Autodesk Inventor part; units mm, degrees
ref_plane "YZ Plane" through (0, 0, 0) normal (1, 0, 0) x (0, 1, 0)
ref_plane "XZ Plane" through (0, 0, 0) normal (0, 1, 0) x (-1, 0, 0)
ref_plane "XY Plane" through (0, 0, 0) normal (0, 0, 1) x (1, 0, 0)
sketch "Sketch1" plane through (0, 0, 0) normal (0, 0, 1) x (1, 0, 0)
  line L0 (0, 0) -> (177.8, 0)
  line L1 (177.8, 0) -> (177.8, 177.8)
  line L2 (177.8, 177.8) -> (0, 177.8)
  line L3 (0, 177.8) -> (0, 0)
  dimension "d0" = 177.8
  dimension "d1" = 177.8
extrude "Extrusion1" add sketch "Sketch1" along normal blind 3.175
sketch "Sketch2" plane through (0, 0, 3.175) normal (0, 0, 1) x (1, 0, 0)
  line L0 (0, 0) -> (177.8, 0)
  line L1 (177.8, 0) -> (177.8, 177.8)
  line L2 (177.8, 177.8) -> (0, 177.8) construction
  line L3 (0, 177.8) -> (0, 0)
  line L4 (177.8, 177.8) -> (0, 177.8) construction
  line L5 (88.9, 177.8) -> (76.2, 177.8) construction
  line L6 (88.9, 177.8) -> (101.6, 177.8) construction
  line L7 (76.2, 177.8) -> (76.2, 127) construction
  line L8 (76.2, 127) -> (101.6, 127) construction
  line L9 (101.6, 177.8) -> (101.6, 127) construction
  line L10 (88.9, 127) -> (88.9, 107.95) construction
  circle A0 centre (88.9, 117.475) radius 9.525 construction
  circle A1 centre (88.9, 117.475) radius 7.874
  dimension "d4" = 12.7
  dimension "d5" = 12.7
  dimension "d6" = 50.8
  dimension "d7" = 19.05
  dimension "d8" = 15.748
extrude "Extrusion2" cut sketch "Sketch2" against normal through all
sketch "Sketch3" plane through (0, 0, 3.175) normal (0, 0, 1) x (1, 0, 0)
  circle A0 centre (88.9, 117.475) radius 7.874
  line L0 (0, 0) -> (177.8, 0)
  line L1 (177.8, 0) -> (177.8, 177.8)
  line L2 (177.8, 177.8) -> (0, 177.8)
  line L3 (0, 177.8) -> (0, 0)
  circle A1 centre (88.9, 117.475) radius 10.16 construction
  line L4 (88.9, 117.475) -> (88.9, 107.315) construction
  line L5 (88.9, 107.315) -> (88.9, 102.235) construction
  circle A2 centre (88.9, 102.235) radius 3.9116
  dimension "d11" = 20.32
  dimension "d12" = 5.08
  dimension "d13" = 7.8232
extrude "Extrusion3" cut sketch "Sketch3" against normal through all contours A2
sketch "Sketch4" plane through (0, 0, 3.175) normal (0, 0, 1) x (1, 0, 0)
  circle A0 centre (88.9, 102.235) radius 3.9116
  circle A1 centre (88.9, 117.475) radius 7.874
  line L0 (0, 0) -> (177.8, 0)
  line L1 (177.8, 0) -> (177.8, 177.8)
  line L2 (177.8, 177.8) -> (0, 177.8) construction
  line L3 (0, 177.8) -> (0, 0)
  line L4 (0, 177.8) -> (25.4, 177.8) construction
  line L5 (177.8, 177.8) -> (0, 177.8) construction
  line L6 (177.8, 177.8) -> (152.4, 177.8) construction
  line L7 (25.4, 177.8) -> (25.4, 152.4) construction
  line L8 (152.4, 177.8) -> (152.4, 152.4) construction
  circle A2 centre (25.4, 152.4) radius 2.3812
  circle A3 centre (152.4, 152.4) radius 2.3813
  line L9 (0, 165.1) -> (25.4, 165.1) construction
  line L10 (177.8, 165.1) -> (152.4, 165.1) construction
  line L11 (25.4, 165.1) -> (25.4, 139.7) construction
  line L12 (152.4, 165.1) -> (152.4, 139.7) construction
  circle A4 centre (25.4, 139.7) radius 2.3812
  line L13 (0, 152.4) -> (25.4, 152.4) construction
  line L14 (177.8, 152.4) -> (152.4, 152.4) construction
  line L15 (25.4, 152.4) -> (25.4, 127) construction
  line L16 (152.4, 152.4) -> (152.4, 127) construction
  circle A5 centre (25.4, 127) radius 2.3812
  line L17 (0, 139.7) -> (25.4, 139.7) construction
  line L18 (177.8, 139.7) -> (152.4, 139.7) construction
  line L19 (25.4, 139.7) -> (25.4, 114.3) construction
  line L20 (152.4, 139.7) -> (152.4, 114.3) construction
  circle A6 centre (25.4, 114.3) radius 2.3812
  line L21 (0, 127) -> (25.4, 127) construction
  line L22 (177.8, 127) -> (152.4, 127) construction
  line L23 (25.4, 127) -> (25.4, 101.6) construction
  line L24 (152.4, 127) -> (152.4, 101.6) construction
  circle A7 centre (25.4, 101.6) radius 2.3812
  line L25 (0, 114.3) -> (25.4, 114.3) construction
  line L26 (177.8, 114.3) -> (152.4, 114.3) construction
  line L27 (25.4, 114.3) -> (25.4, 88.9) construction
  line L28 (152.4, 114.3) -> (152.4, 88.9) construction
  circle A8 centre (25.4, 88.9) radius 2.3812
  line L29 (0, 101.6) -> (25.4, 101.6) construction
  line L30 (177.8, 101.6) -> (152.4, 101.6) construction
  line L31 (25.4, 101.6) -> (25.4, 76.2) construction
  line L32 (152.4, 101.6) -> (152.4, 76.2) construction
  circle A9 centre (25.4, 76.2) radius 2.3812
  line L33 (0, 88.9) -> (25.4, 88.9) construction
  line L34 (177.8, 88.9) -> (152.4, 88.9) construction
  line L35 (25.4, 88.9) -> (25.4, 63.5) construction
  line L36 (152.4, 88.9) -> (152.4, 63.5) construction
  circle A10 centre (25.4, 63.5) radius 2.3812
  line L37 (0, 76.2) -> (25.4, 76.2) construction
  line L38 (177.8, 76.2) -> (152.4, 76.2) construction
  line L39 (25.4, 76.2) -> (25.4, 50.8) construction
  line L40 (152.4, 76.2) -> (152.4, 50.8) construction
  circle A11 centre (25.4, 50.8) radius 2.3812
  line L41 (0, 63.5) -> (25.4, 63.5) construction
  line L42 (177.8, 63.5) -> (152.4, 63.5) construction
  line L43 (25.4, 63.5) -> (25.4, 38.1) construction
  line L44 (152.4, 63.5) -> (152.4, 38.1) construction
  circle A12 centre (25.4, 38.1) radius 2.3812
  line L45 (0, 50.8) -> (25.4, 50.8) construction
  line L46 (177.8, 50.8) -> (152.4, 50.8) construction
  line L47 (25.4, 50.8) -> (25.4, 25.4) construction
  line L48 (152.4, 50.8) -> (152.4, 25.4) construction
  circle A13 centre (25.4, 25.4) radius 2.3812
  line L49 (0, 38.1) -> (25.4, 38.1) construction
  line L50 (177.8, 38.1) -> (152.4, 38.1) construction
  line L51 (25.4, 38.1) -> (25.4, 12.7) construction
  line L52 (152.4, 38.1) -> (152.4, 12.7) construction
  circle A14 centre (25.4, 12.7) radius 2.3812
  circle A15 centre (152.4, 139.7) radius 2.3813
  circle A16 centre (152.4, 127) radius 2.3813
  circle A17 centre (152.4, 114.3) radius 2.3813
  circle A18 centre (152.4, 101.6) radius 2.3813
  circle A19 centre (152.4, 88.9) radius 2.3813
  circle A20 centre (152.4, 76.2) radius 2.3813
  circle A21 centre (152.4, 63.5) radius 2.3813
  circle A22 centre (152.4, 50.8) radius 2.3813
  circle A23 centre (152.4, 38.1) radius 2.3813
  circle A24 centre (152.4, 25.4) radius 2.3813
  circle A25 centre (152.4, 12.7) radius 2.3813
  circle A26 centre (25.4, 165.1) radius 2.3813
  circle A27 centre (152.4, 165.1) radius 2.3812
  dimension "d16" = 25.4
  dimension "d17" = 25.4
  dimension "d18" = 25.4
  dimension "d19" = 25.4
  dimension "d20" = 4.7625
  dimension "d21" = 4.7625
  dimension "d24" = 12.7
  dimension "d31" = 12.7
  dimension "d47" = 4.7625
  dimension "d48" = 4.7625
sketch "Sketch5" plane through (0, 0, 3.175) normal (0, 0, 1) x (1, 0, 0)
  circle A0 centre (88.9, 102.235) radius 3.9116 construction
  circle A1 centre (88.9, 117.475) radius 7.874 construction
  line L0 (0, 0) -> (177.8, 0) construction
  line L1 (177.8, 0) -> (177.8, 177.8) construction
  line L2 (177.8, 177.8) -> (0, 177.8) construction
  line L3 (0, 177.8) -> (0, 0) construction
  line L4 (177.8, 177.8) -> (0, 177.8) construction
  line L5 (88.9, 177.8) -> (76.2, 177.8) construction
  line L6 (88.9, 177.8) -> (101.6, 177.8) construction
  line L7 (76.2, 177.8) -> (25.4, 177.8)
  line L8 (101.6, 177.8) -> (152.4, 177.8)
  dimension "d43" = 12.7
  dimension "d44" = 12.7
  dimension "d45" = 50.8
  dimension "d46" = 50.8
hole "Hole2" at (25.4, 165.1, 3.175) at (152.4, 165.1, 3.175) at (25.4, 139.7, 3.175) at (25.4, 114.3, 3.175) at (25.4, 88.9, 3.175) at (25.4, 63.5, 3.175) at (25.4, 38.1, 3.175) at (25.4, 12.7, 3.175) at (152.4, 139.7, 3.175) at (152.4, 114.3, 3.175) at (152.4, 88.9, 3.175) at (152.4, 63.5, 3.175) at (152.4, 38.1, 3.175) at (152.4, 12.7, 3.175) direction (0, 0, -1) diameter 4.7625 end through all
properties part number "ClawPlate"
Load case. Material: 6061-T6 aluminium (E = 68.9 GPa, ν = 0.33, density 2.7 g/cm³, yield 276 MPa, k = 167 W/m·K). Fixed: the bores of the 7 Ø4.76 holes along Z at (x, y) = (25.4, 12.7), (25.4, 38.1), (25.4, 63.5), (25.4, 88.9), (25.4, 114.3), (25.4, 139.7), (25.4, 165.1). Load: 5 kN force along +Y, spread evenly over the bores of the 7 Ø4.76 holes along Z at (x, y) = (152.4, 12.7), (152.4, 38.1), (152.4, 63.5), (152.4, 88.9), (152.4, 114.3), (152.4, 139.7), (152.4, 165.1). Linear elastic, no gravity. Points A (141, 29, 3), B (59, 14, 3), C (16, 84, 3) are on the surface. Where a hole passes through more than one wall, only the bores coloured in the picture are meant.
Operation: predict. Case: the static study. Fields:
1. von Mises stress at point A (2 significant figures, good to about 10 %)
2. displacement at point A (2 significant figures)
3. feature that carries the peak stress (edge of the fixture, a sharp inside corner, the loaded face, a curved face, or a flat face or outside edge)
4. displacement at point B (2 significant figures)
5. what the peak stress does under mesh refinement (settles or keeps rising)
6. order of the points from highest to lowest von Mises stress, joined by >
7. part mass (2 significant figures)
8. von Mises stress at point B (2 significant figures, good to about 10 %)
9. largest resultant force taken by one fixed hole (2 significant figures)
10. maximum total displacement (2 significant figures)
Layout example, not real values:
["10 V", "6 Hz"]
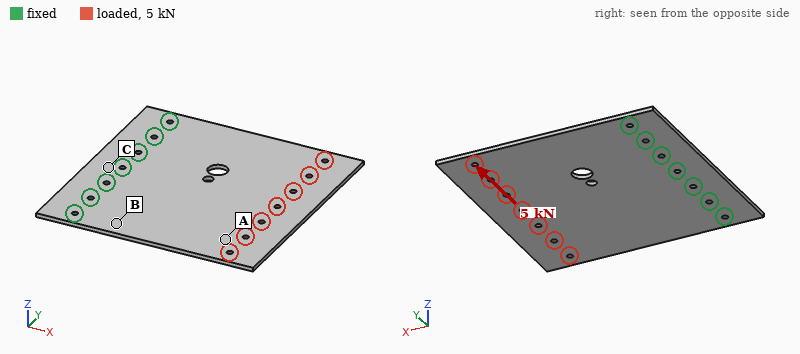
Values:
["14 MPa", "0.086 mm", "edge of the fixture", "0.027 mm", "keeps rising", "B > A > C", "270 g", "26 MPa", "3.2 kN", "0.11 mm"]
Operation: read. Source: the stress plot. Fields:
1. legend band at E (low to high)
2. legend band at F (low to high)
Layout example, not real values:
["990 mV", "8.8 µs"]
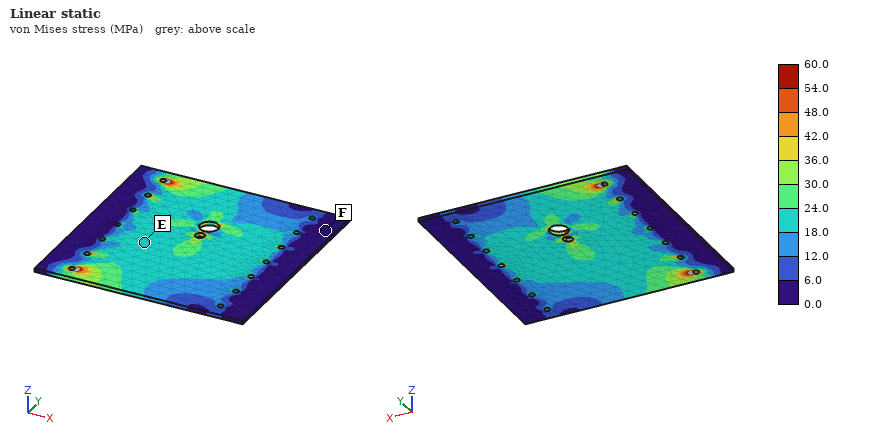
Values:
["18.0 to 24.0 MPa", "0.0 to 6.0 MPa"]
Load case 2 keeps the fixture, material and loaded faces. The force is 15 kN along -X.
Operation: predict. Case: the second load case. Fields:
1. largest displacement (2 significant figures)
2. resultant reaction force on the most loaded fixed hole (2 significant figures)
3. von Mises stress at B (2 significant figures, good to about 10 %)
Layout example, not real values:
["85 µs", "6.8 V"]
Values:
["58 µm", "2.6 kN", "26 MPa"]
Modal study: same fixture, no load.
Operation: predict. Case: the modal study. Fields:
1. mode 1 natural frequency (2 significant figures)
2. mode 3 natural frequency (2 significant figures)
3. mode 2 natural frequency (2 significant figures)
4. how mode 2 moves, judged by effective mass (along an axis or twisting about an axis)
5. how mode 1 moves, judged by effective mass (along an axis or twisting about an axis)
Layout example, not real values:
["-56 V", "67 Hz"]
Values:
["120 Hz", "650 Hz", "250 Hz", "twisting about X", "along Z"]
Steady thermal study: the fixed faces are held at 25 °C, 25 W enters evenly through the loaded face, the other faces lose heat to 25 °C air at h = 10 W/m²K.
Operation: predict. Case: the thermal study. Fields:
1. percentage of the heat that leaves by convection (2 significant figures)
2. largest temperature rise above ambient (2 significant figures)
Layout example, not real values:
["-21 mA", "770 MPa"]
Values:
["33 %", "27 K"]
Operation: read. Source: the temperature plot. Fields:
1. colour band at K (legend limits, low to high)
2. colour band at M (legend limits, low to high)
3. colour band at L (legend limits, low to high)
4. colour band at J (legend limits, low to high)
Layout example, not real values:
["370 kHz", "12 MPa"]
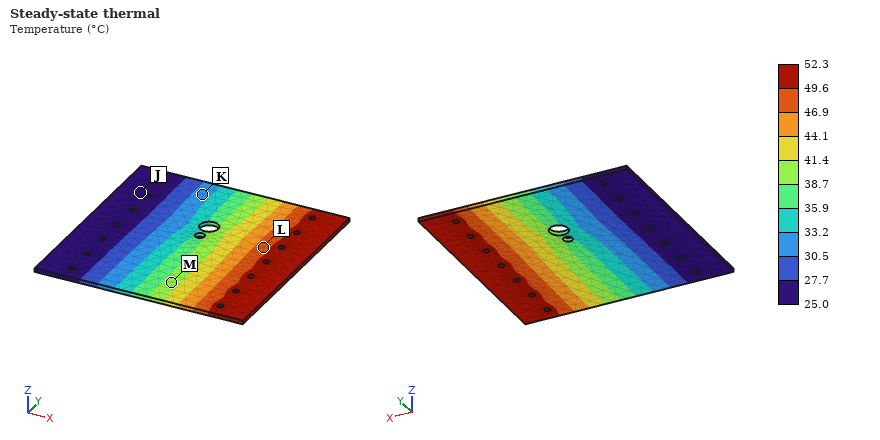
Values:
["30.5 to 33.2 °C", "38.7 to 41.4 °C", "46.9 to 49.6 °C", "25.0 to 27.7 °C"]
